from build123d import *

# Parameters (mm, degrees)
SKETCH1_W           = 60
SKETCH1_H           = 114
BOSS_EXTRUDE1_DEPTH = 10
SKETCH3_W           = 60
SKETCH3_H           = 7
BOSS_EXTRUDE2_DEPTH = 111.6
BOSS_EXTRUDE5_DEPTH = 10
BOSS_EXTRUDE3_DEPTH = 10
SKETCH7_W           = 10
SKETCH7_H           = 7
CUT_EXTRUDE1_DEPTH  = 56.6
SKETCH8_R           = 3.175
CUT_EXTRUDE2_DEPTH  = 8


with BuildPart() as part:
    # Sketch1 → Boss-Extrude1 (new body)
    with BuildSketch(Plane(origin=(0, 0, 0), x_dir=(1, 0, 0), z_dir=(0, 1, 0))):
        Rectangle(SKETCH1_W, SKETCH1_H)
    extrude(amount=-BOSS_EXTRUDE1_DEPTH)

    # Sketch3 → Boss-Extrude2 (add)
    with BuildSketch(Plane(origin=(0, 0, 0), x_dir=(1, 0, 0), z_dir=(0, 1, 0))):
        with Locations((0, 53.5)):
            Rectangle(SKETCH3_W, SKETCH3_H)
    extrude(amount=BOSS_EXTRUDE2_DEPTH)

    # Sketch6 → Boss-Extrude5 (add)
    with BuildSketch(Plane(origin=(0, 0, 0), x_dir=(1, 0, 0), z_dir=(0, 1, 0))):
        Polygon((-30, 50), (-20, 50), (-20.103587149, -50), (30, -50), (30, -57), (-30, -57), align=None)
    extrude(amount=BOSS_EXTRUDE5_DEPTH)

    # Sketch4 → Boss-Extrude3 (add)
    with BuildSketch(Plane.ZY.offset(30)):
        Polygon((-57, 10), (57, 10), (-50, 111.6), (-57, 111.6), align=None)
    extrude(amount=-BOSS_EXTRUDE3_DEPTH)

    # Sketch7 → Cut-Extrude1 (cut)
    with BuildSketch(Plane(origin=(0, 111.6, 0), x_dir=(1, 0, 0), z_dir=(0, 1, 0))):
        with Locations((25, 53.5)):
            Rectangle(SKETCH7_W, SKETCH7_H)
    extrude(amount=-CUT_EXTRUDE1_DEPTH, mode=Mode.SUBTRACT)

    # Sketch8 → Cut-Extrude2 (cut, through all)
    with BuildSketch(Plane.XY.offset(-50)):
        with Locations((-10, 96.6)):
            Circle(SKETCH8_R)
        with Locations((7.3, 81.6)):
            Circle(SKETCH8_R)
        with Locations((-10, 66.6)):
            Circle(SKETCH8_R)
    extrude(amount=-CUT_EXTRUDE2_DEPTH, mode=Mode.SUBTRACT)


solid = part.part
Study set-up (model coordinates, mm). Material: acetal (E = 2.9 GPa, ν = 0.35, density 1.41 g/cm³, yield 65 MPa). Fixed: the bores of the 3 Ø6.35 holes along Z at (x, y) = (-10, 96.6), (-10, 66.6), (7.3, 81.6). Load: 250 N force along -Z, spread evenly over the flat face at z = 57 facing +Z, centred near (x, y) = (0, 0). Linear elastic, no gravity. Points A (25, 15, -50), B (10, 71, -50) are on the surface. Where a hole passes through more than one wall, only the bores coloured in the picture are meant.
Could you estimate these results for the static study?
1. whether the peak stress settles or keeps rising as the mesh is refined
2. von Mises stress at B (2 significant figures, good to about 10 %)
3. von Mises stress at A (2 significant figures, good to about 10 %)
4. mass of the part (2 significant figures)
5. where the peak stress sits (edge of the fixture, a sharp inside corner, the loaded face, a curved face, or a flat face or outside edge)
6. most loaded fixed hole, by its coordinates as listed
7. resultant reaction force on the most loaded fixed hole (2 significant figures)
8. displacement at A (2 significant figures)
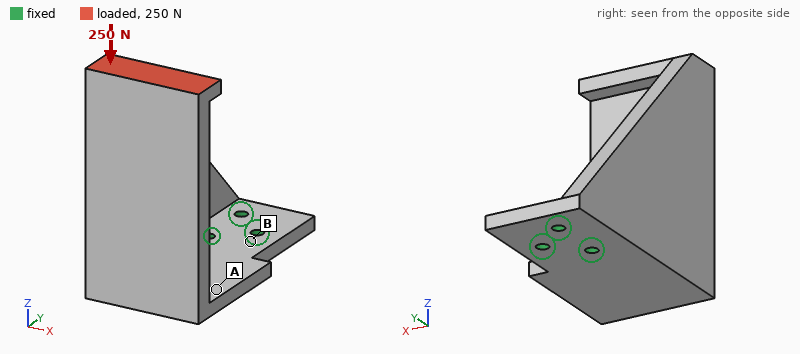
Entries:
keeps rising
6.2 MPa
2.7 MPa
250 g
edge of the fixture
(-10, 66.6)
660 N
0.90 mm
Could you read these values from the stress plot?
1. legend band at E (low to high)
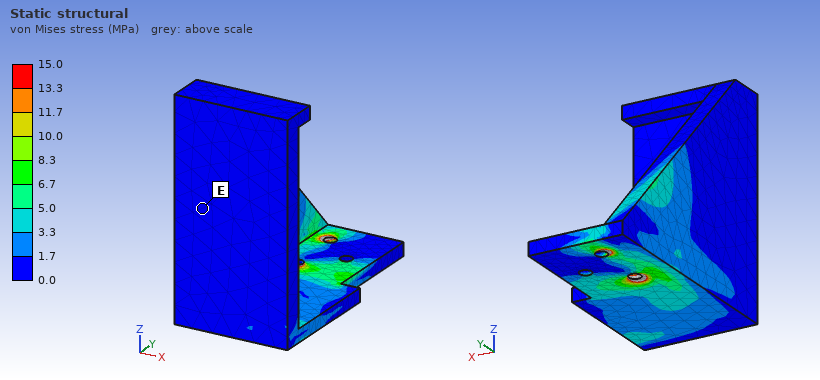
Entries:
0.0 to 1.7 MPa
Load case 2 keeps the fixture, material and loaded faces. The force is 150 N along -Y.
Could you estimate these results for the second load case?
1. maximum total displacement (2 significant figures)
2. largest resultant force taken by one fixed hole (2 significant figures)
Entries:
1.9 mm
480 N
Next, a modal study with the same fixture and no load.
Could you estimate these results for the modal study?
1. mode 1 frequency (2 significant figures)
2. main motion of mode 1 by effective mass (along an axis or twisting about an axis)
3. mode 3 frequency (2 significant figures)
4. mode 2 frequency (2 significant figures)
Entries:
100 Hz
along X
460 Hz
180 Hz
